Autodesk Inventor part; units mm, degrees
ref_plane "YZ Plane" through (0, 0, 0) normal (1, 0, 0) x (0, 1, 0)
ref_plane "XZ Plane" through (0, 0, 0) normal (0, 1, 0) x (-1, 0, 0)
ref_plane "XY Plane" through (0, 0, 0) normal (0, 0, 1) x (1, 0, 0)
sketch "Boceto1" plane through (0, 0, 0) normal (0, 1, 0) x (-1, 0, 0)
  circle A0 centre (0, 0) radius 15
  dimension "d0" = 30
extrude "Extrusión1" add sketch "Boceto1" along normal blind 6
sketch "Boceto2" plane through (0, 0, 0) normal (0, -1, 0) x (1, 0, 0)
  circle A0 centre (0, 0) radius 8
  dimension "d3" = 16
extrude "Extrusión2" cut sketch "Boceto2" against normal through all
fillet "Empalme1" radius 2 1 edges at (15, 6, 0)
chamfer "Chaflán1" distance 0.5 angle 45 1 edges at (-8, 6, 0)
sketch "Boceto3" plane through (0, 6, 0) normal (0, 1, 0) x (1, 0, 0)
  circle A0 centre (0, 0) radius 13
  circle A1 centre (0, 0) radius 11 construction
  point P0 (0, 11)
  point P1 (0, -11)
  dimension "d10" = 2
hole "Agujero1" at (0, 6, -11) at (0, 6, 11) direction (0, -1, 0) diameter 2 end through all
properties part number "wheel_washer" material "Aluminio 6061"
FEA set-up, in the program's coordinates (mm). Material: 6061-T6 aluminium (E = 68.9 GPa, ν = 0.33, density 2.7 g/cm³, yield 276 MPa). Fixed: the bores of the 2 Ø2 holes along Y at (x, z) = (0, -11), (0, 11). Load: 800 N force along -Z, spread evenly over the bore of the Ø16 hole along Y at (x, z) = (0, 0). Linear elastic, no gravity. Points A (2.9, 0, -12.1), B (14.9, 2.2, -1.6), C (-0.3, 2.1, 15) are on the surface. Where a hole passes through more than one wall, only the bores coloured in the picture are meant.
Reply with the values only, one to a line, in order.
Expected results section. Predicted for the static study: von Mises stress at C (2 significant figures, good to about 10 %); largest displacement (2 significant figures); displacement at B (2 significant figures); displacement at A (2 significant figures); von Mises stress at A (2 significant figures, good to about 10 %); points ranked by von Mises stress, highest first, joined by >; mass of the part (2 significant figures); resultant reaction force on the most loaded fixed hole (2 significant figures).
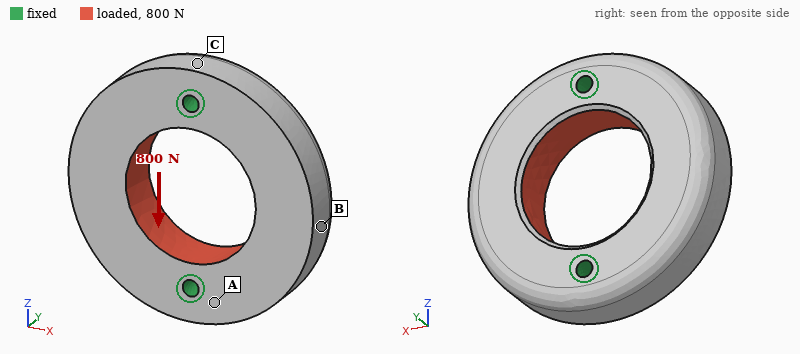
12 MPa
2.4 µm
1.6 µm
0.61 µm
8.2 MPa
C > A > B
7.9 g
400 N
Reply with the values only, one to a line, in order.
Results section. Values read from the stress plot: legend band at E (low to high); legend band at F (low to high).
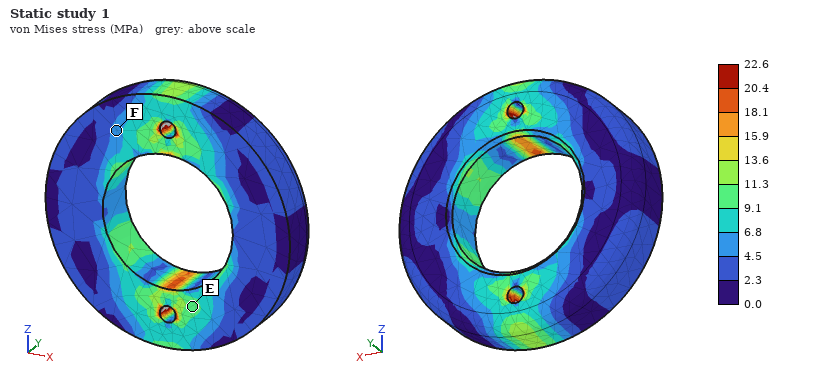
9.1 to 11.3 MPa
4.5 to 6.8 MPa
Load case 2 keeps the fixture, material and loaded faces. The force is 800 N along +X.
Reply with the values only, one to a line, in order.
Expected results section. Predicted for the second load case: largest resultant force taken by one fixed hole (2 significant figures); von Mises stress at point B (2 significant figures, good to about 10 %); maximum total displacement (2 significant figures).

400 N
4.6 MPa
1.8 µm
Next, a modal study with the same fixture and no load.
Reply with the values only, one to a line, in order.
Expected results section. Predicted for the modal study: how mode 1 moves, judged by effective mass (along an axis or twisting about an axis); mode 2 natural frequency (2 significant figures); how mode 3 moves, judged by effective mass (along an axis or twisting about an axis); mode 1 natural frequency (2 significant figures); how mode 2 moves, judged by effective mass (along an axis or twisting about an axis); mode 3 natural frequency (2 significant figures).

twisting about Z
17 kHz
twisting about Y
16 kHz
along Y
28 kHz
